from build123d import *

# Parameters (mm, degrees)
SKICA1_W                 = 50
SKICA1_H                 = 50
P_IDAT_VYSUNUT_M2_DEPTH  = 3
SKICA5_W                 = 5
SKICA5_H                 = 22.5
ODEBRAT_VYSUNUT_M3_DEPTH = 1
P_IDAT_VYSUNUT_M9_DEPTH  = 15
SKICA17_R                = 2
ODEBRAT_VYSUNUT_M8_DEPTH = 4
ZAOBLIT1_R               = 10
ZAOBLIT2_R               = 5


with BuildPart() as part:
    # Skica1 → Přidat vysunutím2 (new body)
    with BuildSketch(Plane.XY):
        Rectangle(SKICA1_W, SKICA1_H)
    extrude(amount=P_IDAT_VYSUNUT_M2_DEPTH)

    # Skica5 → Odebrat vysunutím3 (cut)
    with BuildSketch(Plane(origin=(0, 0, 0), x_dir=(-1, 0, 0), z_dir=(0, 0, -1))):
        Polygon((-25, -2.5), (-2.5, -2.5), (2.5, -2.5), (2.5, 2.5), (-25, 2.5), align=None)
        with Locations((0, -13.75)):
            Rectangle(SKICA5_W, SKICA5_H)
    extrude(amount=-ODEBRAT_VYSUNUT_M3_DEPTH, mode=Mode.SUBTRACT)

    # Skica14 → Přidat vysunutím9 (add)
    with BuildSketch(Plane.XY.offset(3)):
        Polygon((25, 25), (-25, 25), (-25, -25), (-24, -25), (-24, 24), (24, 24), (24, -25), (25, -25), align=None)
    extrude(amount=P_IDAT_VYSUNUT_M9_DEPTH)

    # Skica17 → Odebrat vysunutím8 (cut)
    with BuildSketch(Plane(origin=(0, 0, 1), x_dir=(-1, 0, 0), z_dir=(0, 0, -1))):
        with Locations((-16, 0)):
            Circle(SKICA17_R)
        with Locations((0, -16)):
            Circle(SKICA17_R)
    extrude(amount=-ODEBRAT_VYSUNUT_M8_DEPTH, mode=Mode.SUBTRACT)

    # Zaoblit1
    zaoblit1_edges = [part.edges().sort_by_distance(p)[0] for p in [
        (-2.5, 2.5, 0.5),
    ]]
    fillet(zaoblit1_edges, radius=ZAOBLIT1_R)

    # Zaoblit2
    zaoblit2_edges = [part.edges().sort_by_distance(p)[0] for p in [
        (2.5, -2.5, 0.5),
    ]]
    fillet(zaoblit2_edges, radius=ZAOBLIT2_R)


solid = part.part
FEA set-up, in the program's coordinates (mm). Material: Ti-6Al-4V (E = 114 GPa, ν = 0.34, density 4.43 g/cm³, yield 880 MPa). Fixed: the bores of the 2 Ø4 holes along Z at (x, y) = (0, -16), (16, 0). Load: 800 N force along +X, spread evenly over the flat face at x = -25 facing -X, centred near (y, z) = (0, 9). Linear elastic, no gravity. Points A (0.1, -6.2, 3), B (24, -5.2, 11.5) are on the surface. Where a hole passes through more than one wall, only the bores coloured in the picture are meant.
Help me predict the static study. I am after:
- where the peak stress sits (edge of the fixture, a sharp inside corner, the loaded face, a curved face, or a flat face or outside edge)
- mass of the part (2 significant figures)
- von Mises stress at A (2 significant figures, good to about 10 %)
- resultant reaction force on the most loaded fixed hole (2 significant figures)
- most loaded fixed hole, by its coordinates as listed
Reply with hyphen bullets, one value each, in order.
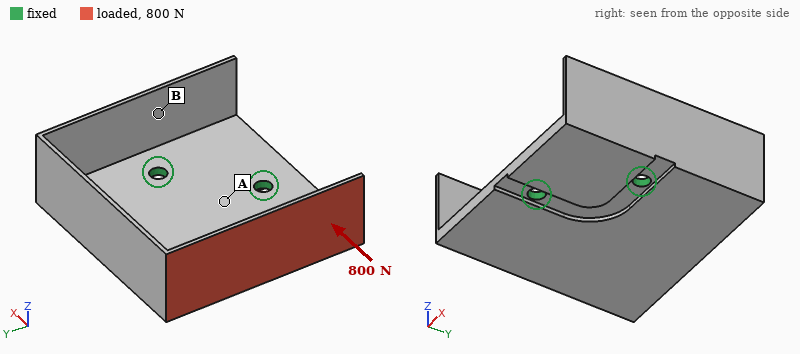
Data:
- the loaded face
- 42 g
- 90 MPa
- 590 N
- (16, 0)
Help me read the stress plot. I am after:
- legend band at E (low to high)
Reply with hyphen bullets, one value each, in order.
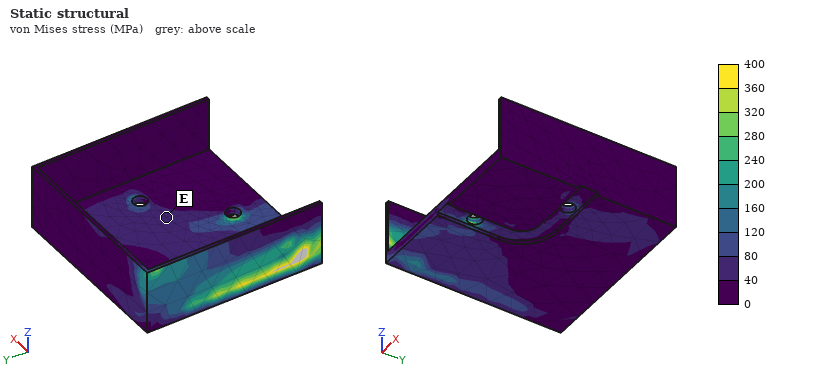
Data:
- 40 to 80 MPa
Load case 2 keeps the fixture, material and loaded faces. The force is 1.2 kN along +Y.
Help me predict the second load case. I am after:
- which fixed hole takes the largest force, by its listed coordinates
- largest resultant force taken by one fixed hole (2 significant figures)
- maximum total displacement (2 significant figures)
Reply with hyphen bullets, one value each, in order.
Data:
- (0, -16)
- 2.1 kN
- 0.63 mm
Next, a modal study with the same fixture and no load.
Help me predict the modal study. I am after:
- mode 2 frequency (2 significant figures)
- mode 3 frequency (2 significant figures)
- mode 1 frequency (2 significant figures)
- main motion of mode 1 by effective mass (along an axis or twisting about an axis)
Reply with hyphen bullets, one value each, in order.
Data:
- 2600 Hz
- 3300 Hz
- 1200 Hz
- along Z
